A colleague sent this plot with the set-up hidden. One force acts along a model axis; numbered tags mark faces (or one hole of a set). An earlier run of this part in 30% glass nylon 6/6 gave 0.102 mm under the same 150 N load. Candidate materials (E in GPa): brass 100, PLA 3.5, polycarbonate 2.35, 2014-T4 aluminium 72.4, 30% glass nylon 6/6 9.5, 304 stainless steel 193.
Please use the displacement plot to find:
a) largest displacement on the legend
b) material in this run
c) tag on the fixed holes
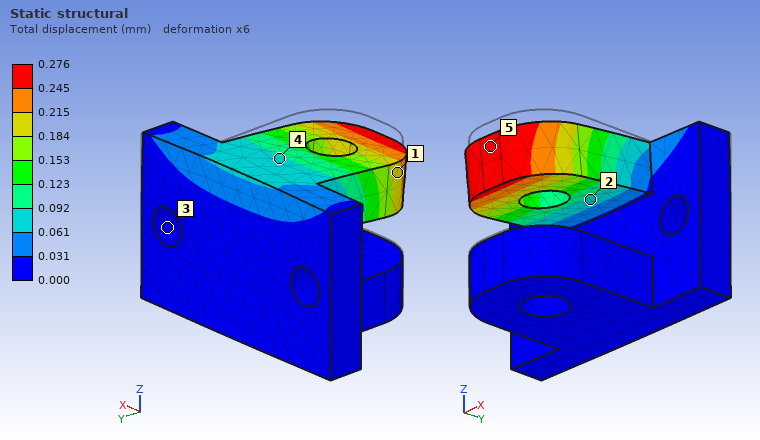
0.276 mm
PLA
3
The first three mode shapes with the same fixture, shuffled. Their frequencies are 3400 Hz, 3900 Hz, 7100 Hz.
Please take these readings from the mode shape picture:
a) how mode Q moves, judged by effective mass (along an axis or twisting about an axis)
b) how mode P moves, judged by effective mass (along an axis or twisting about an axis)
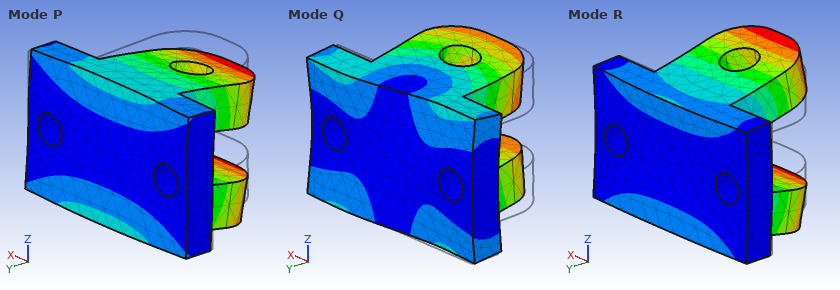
along X
along Z
